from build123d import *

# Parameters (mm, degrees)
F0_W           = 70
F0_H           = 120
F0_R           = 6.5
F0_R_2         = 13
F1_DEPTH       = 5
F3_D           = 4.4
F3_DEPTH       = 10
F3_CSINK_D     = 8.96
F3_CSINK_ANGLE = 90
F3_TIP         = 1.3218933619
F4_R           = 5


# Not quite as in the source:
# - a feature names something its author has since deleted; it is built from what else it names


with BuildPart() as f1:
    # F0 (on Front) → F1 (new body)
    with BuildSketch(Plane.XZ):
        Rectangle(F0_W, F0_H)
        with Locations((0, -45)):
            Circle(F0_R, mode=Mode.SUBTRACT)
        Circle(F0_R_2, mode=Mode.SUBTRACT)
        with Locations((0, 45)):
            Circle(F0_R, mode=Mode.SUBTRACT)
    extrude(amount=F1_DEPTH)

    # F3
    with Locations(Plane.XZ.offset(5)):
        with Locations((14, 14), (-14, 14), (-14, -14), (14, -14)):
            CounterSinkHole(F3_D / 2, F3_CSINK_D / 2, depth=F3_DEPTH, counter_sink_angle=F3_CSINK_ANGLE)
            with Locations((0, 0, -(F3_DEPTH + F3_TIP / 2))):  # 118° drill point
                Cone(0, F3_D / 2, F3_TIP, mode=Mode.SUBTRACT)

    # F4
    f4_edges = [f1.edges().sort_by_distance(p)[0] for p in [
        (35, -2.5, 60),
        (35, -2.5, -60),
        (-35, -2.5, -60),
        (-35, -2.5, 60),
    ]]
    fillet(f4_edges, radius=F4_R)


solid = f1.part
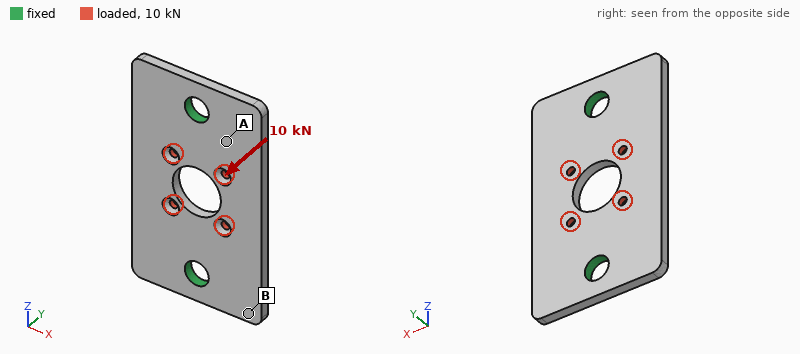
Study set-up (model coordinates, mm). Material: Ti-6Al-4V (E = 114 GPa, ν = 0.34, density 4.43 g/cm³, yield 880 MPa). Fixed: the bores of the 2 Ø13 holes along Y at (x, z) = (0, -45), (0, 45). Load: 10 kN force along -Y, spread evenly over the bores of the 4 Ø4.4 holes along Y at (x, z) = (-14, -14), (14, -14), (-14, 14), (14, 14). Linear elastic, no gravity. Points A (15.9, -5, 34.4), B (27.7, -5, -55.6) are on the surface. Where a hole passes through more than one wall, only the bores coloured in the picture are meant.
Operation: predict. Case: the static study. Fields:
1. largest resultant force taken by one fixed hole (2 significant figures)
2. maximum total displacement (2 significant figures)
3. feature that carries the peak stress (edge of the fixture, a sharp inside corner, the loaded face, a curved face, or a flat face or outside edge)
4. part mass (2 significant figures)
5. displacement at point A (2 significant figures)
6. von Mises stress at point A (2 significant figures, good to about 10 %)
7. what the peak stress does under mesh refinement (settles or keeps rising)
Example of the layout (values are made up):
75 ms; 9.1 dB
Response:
5.0 kN; 0.45 mm; edge of the fixture; 170 g; 0.088 mm; 170 MPa; keeps rising
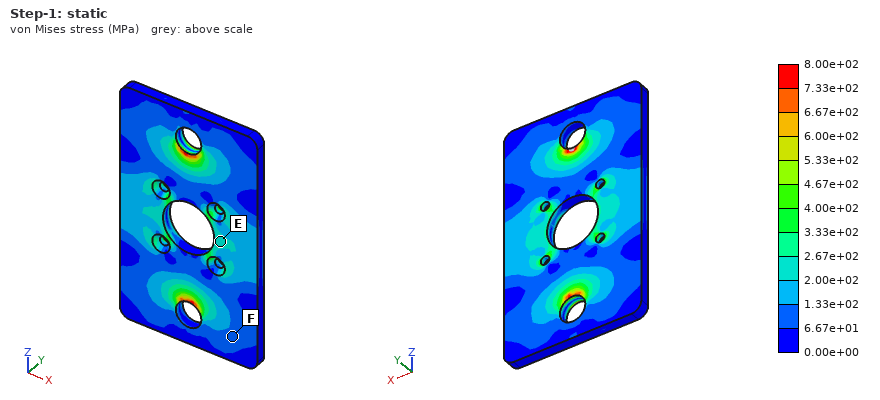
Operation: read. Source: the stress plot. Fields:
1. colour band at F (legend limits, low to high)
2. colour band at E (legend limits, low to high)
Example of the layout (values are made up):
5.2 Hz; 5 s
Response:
6.67e+01 to 1.33e+02 MPa; 2.00e+02 to 2.67e+02 MPa
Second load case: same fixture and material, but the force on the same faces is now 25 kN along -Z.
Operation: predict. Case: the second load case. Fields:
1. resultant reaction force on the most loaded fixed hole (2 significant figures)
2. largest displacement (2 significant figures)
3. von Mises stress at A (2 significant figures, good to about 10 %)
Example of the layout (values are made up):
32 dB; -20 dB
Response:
13 kN; 30 µm; 40 MPa
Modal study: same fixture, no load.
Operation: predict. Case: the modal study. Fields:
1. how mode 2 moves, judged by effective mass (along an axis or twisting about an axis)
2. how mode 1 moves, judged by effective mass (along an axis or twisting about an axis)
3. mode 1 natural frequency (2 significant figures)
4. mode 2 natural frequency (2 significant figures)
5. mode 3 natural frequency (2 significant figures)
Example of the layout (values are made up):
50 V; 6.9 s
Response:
along Y; twisting about Z; 2600 Hz; 2900 Hz; 4600 Hz
